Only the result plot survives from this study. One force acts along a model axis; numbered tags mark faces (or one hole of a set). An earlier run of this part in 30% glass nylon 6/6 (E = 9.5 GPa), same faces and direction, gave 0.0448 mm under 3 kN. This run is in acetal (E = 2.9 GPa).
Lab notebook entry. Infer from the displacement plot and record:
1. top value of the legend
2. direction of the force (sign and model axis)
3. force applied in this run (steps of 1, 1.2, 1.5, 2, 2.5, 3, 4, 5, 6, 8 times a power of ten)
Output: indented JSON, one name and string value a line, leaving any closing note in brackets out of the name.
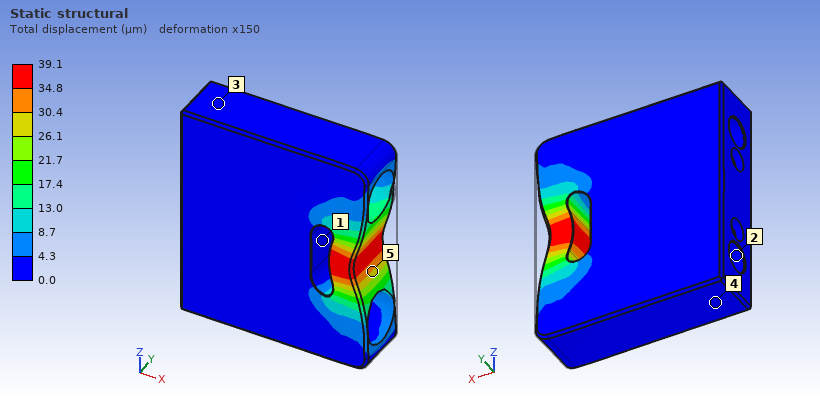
{
  "top value of the legend": "39.1 µm",
  "direction of the force": "-X",
  "force applied in this run": "800 N"
}
